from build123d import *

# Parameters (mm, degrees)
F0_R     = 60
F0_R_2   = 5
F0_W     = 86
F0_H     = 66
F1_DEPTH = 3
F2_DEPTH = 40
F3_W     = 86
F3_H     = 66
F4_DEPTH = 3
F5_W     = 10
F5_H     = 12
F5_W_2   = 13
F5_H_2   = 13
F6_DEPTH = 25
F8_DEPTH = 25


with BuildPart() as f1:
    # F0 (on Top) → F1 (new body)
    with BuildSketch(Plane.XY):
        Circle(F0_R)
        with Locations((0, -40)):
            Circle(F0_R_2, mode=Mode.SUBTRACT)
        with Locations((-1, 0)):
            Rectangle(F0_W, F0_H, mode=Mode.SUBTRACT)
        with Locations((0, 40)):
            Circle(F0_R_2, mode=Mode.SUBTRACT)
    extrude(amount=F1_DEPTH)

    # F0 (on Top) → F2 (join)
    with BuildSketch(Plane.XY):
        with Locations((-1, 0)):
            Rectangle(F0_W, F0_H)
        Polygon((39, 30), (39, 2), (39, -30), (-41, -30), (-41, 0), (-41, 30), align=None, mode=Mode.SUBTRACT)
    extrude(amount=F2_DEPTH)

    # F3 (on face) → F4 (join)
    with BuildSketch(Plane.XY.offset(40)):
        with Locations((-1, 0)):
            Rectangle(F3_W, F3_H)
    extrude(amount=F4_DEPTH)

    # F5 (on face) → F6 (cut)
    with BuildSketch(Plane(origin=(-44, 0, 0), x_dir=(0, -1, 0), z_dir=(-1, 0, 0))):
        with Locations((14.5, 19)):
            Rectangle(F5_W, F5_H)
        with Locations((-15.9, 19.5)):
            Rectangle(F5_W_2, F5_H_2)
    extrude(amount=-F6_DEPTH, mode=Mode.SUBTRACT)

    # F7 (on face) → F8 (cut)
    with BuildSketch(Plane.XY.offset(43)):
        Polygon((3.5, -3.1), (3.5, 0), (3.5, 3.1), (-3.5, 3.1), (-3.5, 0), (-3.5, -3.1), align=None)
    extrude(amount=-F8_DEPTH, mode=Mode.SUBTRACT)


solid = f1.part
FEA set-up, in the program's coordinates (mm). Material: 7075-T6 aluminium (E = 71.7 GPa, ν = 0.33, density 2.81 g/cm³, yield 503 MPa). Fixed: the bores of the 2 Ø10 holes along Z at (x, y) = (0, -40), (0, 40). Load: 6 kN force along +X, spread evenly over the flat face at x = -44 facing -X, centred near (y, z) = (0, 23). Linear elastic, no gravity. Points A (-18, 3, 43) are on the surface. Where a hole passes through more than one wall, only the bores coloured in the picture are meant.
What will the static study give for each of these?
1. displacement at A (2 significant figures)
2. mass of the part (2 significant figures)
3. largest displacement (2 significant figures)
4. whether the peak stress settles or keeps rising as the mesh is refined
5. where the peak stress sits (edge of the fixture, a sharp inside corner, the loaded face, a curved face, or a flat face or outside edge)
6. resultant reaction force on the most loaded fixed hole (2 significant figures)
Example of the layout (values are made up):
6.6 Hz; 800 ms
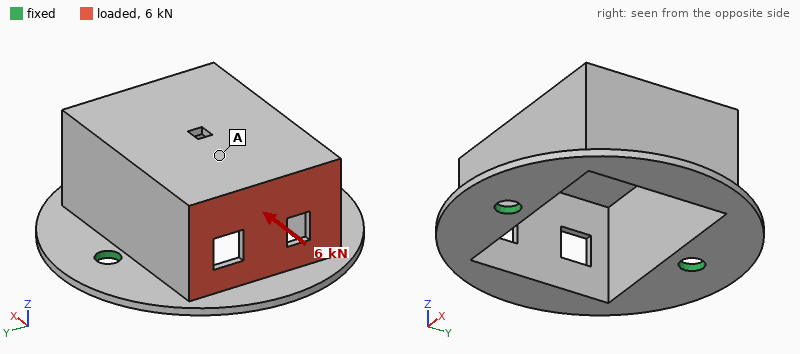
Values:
0.88 mm; 190 g; 1.3 mm; keeps rising; edge of the fixture; 3.1 kN
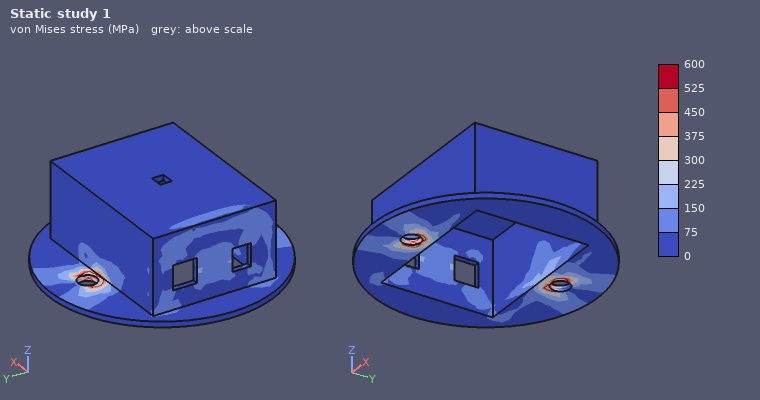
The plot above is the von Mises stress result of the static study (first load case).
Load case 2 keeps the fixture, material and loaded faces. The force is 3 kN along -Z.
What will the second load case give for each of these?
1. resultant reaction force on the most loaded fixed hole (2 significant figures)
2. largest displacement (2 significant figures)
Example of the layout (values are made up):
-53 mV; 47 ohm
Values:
1.6 kN; 1.2 mm
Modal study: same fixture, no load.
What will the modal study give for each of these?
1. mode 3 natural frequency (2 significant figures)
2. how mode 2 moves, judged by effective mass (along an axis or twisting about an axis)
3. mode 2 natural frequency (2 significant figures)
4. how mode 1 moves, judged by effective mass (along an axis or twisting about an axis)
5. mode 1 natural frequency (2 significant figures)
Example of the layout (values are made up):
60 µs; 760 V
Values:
3200 Hz; along Y; 3000 Hz; along X; 760 Hz
